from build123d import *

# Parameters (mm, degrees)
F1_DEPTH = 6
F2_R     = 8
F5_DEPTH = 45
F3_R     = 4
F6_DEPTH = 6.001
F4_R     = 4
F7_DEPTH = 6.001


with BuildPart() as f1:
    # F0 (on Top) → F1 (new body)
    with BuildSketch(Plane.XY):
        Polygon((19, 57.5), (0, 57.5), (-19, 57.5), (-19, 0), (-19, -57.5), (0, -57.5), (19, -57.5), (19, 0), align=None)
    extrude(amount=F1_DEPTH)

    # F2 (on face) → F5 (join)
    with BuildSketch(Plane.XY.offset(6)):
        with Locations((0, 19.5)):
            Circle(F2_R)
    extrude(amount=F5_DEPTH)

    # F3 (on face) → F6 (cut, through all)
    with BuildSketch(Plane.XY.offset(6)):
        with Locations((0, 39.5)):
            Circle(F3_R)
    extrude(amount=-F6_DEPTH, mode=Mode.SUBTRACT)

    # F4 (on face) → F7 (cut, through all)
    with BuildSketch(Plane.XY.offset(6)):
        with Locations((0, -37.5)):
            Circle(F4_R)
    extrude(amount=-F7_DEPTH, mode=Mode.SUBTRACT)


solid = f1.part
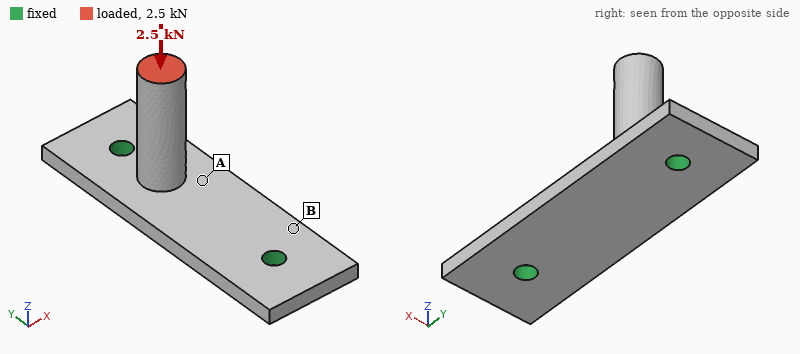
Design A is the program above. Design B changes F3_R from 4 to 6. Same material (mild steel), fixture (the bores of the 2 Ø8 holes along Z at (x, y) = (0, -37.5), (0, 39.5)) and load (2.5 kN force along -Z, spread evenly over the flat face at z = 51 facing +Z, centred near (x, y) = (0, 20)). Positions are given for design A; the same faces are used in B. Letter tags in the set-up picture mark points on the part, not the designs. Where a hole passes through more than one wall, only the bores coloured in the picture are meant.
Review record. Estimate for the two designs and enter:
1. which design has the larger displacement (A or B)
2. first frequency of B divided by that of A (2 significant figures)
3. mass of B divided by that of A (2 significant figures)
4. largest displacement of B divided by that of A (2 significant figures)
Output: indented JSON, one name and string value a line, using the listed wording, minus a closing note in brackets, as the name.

{
  "which design has the larger displacement": "A",
  "first frequency of B divided by that of A": "1.1",
  "mass of B divided by that of A": "0.99",
  "largest displacement of B divided by that of A": "0.88"
}
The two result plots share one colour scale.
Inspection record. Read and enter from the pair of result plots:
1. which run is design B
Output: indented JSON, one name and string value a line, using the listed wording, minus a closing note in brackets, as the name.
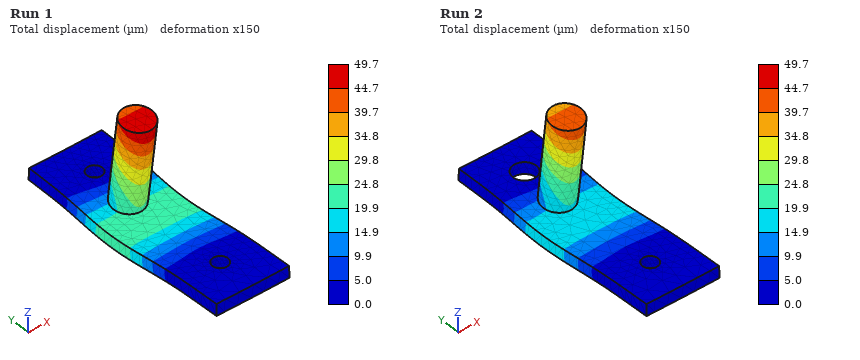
{
  "which run is design B": "Run 2"
}
